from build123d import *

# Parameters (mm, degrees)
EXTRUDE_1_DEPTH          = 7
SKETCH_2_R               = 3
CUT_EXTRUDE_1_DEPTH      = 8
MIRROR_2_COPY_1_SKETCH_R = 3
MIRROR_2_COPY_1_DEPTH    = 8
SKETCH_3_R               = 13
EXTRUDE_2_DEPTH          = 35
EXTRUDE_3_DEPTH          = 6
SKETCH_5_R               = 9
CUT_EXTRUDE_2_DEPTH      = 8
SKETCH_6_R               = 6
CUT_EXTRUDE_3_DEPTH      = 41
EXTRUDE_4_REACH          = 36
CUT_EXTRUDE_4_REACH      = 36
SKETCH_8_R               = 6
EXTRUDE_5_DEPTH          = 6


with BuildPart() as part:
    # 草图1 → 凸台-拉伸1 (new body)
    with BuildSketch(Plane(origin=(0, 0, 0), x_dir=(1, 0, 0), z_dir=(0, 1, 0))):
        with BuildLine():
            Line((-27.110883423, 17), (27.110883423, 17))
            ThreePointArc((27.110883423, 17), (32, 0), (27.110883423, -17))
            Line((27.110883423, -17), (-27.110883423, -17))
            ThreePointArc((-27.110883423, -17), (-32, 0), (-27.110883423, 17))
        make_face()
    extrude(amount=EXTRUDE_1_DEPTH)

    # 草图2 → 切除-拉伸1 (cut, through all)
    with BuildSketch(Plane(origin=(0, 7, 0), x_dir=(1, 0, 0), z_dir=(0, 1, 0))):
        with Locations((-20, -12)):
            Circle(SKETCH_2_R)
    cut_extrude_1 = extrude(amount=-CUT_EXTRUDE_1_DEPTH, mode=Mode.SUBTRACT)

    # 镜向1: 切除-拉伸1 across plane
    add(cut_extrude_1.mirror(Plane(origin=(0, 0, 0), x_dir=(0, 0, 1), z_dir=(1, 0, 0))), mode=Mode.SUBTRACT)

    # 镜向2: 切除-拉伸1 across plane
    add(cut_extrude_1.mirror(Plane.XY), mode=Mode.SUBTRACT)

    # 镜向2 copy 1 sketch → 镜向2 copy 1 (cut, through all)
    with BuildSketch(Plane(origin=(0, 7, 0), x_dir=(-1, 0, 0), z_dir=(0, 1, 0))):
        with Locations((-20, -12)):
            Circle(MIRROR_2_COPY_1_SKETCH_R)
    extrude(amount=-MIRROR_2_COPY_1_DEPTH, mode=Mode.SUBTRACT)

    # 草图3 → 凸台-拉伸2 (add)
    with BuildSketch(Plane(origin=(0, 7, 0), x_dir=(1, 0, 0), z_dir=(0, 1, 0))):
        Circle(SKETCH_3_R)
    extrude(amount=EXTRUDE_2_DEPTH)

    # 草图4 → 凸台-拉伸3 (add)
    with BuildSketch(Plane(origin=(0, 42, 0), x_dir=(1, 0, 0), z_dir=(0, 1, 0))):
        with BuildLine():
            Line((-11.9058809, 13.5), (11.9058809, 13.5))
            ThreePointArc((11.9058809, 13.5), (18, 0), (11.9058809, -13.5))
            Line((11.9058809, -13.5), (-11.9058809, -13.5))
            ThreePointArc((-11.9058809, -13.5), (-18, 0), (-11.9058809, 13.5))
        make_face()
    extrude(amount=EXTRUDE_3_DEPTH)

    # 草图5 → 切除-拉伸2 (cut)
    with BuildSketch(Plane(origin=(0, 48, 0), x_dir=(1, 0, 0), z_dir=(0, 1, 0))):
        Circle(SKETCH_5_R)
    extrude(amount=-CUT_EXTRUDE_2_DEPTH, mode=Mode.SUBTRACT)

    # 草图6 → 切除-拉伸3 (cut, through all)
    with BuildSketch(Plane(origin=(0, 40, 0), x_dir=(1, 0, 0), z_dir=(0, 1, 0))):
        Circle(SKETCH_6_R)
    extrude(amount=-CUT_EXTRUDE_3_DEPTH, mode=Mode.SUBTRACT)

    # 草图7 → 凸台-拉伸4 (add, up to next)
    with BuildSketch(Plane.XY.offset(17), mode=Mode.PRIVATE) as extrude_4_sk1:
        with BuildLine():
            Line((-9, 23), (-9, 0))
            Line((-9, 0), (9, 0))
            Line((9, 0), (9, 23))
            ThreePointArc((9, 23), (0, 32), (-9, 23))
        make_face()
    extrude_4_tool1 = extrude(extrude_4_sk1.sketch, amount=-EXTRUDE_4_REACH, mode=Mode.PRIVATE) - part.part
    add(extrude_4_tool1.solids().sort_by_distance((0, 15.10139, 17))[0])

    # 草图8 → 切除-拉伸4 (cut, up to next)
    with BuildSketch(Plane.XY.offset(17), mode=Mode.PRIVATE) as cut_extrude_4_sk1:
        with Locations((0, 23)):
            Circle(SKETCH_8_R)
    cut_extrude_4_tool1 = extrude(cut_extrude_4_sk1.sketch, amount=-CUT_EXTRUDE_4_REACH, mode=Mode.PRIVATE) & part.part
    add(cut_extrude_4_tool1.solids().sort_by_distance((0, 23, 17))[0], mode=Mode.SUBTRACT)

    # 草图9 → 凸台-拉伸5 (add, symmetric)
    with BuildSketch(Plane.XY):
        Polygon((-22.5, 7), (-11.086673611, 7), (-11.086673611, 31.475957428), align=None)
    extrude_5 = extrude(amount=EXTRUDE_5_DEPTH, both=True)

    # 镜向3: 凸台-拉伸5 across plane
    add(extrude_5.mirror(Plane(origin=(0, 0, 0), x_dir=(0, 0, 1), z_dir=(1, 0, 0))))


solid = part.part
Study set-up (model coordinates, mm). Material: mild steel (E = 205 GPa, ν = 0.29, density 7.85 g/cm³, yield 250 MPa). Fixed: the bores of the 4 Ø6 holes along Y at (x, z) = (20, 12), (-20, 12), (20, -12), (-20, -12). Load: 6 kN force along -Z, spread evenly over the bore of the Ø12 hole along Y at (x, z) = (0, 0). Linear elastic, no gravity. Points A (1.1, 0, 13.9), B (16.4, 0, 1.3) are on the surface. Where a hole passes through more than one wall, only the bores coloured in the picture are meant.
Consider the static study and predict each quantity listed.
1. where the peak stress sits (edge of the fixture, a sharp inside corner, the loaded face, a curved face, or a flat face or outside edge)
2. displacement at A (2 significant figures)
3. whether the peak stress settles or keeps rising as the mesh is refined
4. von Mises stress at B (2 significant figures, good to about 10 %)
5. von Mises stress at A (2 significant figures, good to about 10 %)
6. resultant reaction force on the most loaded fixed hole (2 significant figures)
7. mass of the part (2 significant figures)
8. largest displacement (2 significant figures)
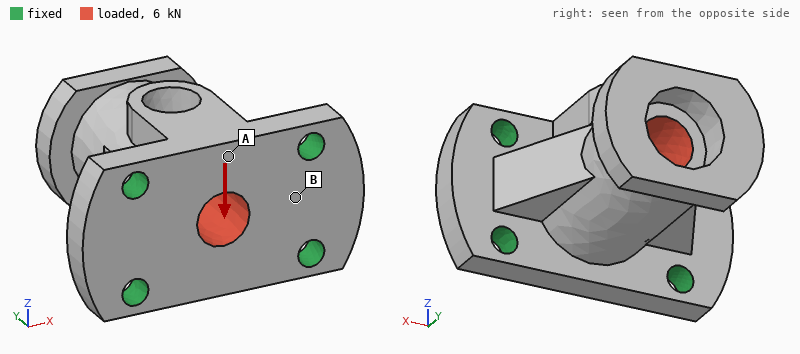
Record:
edge of the fixture
5.8 µm
keeps rising
13 MPa
27 MPa
2.9 kN
270 g
29 µm
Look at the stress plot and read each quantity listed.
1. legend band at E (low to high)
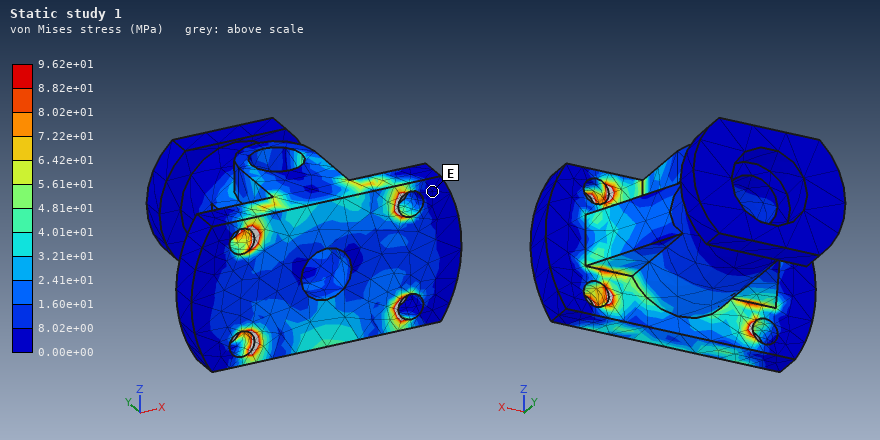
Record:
0.00e+00 to 8.02e+00 MPa
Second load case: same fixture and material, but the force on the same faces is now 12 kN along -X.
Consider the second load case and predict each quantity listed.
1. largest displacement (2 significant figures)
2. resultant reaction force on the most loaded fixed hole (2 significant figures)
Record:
19 µm
4.1 kN
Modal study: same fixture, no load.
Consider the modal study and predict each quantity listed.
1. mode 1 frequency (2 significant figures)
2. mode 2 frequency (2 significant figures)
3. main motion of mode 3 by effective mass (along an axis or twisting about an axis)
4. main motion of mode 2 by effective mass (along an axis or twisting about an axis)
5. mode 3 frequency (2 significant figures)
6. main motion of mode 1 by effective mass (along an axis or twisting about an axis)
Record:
5500 Hz
9200 Hz
along Y
along X
15 kHz
along Z
